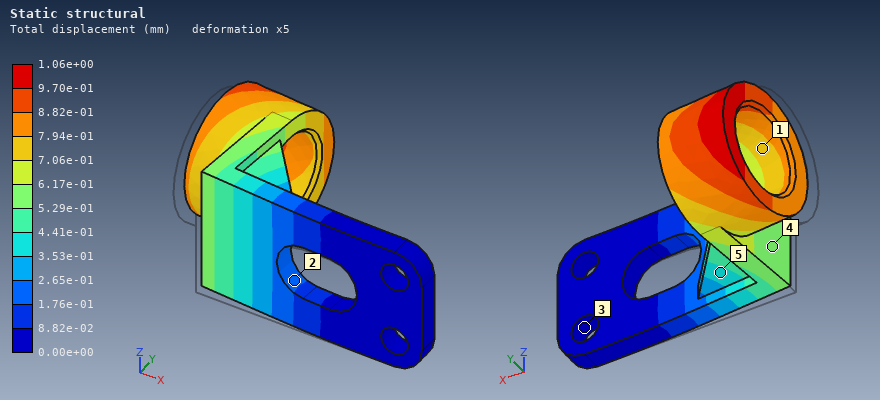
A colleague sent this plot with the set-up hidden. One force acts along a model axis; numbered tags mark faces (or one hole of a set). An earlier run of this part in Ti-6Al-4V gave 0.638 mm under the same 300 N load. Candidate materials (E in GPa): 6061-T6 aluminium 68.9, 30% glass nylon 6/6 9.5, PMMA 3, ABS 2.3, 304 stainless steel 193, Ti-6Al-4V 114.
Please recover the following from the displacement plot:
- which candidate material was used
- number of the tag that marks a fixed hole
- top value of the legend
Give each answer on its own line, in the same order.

6061-T6 aluminium
3
1.06e+00 mm
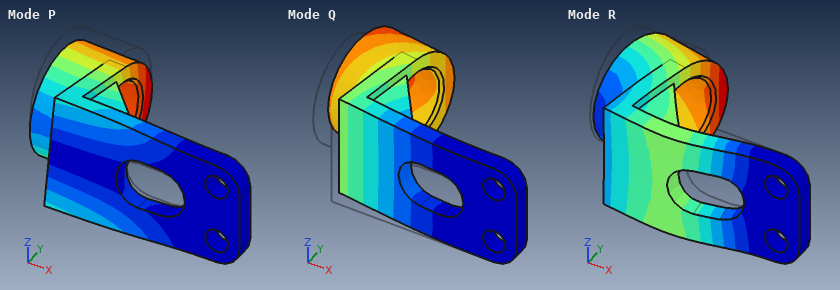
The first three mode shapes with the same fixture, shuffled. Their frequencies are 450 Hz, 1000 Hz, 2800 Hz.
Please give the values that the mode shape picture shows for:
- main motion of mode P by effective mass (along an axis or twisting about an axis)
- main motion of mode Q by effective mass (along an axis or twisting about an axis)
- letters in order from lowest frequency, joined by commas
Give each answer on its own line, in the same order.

along Z
along Y
Q, P, R
